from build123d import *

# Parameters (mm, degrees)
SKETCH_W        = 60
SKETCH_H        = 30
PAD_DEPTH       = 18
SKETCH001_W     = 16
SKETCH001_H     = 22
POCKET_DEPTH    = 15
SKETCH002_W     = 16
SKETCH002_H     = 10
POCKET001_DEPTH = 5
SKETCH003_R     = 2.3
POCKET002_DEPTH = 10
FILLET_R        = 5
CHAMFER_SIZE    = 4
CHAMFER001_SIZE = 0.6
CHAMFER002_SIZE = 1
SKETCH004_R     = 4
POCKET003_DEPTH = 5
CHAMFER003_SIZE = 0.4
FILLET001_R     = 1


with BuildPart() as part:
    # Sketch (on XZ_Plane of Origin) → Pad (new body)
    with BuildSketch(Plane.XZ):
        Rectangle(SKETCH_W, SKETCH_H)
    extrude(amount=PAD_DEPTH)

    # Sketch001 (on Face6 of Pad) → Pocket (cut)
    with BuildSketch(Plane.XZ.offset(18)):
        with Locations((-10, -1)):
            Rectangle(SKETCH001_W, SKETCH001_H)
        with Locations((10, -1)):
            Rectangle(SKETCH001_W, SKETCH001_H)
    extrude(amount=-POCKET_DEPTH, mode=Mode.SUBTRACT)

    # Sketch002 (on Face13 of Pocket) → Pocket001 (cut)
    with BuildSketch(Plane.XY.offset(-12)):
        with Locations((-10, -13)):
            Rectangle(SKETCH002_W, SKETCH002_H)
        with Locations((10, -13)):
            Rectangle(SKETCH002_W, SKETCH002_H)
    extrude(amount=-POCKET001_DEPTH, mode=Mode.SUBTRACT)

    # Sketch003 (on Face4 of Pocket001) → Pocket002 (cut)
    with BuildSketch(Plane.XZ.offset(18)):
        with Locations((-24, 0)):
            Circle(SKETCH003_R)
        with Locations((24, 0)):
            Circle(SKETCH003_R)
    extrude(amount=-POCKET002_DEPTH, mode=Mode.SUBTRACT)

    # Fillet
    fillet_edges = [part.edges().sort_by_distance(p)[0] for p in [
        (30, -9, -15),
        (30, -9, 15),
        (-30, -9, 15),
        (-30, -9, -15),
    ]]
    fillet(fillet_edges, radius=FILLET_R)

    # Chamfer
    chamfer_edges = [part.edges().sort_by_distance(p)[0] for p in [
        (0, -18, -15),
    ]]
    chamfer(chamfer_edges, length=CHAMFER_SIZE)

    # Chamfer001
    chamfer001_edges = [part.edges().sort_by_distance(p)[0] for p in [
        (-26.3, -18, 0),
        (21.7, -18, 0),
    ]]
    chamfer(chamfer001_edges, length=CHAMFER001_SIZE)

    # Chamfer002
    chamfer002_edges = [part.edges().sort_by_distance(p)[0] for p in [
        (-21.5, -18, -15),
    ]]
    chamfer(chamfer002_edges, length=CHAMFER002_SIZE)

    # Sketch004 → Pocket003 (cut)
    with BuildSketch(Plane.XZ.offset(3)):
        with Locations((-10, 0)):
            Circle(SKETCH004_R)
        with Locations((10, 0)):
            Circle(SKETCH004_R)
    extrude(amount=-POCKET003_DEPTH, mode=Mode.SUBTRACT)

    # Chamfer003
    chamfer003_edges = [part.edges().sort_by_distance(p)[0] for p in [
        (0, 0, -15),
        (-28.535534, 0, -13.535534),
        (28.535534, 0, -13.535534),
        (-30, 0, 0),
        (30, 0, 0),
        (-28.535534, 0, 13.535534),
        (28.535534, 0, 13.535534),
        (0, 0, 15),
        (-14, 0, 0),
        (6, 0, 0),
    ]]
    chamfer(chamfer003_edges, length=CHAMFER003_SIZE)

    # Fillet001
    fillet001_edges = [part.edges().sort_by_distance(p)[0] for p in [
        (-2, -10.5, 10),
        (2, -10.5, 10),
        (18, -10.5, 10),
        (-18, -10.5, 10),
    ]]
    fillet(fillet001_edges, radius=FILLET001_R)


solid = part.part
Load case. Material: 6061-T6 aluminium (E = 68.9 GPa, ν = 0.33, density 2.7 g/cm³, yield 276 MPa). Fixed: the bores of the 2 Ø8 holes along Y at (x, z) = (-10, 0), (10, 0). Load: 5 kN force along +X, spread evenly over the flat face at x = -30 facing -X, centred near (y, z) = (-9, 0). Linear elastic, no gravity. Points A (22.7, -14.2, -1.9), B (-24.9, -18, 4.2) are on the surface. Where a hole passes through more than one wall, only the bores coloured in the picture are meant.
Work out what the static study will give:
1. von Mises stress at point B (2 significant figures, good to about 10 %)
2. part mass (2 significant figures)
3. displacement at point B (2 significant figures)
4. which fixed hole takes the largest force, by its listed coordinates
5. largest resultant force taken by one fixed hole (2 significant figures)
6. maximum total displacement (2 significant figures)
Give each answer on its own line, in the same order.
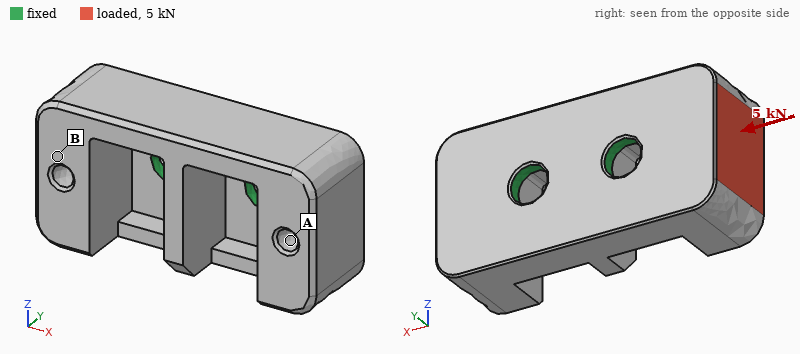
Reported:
50 MPa
53 g
0.096 mm
(-10, 0)
3.3 kN
0.12 mm
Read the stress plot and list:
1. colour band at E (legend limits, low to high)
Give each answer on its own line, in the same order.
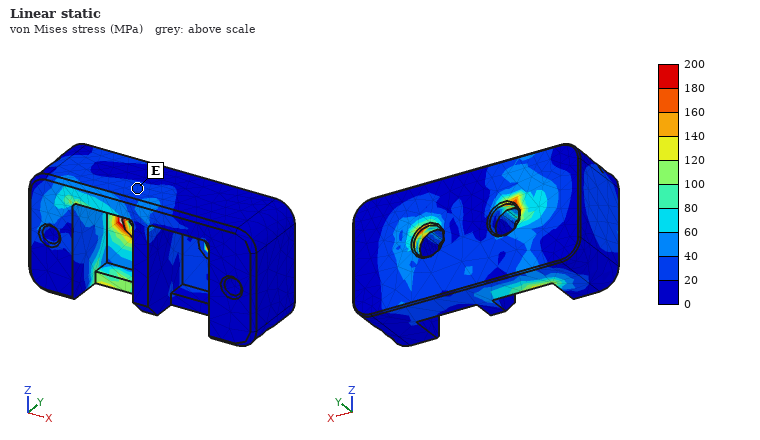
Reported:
20 to 40 MPa
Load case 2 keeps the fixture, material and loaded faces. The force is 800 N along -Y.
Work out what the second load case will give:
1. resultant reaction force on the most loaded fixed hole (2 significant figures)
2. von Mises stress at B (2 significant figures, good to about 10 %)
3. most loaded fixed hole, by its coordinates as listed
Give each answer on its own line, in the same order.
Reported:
1.3 kN
16 MPa
(-10, 0)
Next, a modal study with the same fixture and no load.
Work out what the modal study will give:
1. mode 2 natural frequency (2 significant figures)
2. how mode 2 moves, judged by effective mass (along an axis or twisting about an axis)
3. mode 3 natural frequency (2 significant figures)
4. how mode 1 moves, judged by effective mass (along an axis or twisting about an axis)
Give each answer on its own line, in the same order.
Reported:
5200 Hz
along X
7400 Hz
along Z
